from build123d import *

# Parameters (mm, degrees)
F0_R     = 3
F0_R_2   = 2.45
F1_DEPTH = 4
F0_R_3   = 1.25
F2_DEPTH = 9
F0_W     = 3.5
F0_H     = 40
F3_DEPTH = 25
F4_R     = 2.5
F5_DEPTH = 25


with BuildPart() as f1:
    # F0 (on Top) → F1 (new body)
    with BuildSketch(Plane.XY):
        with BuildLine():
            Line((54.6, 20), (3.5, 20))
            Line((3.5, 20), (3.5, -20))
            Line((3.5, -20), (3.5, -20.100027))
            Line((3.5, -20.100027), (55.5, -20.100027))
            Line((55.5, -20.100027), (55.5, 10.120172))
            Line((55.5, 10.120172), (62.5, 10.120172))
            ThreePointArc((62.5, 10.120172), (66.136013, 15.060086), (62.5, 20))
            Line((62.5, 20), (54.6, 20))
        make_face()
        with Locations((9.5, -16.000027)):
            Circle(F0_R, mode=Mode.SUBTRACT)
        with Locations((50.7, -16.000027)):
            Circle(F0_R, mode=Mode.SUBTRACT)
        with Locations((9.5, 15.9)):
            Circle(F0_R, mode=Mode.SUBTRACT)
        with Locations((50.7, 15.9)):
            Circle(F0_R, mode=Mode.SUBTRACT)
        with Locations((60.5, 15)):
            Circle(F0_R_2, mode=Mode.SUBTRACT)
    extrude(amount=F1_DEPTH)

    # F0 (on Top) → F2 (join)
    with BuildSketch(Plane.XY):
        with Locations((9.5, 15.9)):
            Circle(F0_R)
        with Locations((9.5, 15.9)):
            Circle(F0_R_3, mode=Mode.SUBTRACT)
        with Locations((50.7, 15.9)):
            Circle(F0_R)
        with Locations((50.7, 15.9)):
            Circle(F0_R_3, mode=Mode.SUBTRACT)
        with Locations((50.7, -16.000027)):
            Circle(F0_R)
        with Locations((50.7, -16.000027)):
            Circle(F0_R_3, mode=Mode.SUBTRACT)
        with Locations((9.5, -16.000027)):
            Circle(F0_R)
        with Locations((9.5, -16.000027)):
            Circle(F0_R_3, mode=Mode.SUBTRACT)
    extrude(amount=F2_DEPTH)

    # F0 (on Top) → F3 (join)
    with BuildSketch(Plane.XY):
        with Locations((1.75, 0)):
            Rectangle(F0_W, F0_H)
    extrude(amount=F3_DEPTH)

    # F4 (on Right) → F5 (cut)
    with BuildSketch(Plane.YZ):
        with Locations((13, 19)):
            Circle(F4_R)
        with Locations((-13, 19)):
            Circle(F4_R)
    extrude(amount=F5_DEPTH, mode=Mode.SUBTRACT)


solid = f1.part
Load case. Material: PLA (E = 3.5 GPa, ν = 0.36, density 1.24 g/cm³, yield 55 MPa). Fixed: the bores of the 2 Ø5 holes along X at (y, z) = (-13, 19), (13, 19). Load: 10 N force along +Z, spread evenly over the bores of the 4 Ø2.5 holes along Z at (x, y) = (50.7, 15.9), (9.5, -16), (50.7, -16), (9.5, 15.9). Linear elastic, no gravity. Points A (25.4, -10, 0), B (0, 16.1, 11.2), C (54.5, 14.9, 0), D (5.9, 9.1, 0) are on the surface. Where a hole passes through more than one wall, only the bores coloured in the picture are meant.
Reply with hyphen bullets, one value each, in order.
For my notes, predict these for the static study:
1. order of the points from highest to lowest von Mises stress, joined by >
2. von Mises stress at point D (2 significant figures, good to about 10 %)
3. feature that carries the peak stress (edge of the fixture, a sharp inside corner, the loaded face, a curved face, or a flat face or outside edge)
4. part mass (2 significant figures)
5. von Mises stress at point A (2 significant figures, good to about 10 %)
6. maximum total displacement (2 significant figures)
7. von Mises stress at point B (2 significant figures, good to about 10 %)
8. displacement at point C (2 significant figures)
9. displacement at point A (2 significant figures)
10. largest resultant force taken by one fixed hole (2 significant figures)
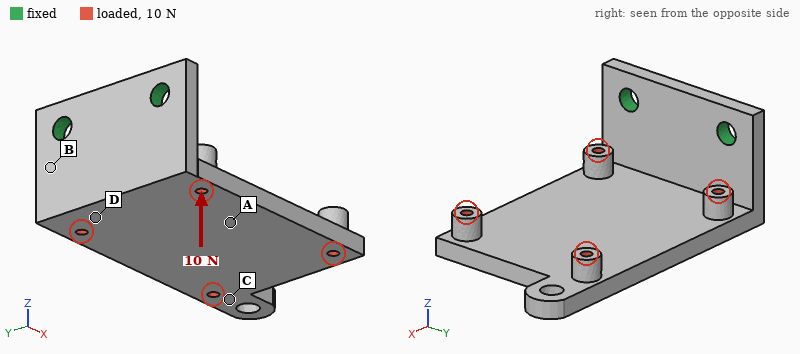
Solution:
- B > D > A > C
- 2.1 MPa
- a flat face or outside edge
- 15 g
- 1.1 MPa
- 0.89 mm
- 3.4 MPa
- 0.71 mm
- 0.28 mm
- 5.5 N
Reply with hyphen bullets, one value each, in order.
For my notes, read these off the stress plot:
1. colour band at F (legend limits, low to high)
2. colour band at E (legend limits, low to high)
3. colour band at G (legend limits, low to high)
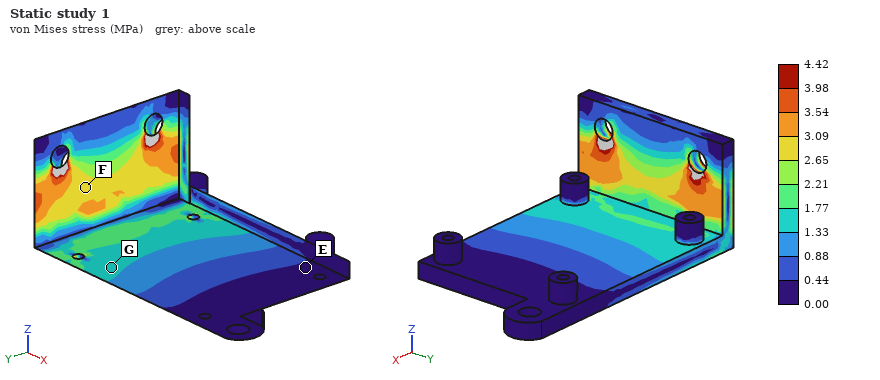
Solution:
- 2.65 to 3.09 MPa
- 0.00 to 0.44 MPa
- 1.33 to 1.77 MPa
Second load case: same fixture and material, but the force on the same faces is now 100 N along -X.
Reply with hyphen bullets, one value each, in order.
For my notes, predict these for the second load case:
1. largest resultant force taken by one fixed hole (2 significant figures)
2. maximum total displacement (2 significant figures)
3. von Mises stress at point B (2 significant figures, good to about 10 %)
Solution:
- 50 N
- 0.83 mm
- 8.7 MPa
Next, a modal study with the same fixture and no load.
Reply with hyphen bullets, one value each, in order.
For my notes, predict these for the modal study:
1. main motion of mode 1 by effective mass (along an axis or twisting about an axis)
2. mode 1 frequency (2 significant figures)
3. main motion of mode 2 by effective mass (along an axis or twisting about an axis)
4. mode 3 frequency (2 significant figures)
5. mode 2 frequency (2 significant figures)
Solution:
- along Z
- 210 Hz
- along Y
- 940 Hz
- 520 Hz
